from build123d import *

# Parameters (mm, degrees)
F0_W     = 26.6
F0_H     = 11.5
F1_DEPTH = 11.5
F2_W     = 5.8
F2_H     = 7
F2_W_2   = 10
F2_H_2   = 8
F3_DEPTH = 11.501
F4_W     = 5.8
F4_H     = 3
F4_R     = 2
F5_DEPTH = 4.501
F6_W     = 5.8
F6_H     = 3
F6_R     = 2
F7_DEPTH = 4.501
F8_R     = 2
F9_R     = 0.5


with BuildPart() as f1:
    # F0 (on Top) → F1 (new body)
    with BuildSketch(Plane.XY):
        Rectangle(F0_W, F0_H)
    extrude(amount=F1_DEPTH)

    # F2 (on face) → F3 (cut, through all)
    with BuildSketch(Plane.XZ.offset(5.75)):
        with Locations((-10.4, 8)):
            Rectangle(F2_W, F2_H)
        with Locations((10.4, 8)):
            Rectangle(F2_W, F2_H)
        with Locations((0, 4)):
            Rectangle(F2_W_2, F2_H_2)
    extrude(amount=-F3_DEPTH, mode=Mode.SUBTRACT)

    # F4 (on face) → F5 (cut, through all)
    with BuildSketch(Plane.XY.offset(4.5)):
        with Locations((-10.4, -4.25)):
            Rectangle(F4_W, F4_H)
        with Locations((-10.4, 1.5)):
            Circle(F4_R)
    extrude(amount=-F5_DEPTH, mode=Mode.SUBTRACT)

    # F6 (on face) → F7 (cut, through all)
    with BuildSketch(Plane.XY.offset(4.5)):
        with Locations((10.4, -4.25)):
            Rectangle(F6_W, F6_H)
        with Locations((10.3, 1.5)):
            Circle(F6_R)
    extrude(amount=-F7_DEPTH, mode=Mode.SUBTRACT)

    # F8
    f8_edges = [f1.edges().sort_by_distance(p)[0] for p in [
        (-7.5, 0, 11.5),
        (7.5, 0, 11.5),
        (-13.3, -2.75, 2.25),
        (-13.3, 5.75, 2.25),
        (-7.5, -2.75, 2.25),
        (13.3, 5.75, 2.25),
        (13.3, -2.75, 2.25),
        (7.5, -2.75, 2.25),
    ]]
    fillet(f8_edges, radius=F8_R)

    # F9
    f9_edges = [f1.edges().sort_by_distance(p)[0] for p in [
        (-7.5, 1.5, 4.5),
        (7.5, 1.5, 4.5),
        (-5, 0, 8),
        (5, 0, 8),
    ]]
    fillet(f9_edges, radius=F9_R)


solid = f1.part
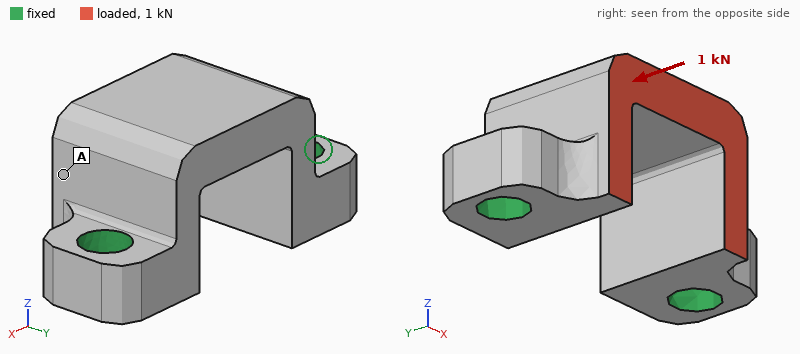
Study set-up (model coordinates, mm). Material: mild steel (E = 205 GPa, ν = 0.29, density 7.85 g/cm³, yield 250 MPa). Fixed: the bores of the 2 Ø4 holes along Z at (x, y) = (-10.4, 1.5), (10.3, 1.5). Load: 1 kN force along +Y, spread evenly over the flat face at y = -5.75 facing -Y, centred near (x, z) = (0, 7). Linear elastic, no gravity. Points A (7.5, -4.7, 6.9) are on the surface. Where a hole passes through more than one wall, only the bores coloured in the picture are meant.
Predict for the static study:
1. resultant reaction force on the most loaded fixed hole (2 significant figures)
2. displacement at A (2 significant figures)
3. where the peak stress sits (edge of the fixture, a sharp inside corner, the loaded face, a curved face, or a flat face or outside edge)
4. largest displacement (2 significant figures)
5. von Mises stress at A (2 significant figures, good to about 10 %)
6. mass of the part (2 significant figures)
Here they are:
500 N
4.3 µm
edge of the fixture
7.4 µm
22 MPa
11 g
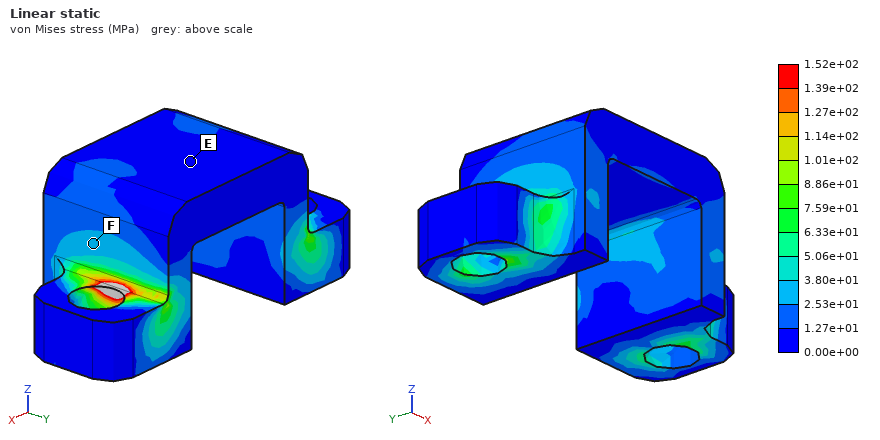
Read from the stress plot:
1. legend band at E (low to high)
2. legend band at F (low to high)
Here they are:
0.00e+00 to 1.27e+01 MPa
2.53e+01 to 3.80e+01 MPa
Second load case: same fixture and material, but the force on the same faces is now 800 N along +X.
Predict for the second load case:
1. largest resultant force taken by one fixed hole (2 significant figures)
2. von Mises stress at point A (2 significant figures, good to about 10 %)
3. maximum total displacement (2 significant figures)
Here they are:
470 N
40 MPa
6.2 µm
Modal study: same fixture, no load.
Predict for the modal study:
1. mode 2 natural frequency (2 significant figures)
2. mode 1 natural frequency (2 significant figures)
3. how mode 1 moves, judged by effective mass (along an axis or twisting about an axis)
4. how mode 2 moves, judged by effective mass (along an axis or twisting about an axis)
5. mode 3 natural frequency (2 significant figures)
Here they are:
31 kHz
24 kHz
along Y
along X
39 kHz
